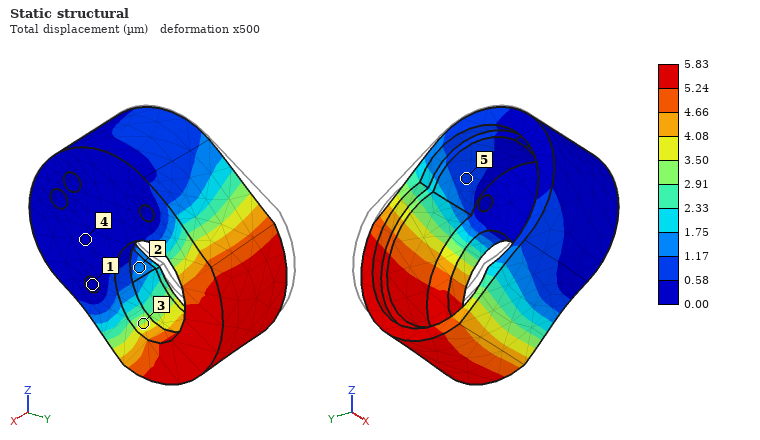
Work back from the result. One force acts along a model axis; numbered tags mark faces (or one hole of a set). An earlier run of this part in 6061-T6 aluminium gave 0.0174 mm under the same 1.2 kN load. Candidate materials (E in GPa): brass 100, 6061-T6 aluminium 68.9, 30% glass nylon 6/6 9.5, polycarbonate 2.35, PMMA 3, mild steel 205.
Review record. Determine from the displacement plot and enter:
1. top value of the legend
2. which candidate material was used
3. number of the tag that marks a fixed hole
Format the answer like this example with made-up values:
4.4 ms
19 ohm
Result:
5.83 µm
mild steel
1
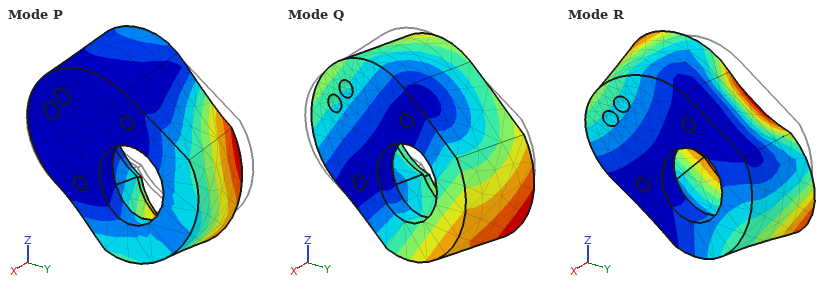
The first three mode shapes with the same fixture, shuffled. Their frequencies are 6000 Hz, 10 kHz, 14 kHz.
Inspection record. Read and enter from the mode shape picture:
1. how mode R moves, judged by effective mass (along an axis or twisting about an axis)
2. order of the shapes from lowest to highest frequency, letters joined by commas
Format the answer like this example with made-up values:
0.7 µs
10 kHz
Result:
along X
Q, P, R
